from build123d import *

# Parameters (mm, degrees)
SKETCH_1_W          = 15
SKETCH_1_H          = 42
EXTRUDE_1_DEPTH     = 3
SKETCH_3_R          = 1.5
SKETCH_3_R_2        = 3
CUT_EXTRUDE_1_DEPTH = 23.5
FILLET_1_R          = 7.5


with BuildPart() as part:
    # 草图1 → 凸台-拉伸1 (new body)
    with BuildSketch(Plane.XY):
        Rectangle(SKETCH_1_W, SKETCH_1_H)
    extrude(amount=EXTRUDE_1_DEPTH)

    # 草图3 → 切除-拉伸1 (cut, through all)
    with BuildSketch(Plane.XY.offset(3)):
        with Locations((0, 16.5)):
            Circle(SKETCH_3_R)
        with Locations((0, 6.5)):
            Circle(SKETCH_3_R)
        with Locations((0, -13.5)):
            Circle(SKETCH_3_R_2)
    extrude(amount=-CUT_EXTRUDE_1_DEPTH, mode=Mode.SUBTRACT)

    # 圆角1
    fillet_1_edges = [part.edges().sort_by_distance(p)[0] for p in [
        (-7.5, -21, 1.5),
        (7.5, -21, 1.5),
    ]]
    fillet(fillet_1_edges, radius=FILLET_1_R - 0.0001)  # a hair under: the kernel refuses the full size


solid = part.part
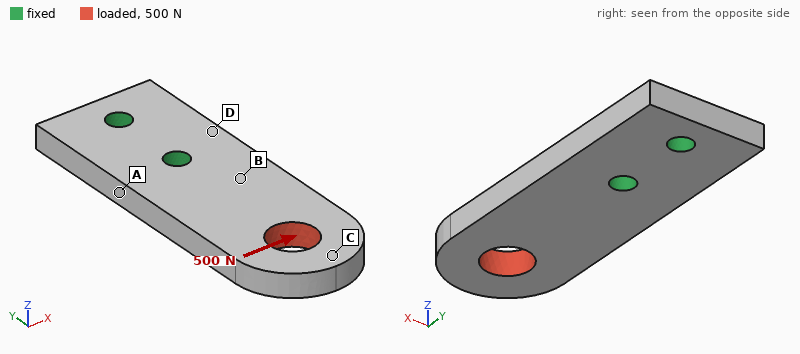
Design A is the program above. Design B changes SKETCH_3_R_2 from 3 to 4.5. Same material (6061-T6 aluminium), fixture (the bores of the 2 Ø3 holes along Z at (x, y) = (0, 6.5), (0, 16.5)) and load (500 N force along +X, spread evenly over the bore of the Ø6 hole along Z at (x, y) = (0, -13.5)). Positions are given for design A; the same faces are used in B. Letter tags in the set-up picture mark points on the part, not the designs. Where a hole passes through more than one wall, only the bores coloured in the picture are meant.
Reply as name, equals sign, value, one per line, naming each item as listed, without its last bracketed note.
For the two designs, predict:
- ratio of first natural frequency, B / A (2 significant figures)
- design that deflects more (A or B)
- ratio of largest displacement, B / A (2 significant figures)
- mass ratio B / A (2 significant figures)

ratio of first natural frequency, B / A = 1.1
design that deflects more = B
ratio of largest displacement, B / A = 1.2
mass ratio B / A = 0.94
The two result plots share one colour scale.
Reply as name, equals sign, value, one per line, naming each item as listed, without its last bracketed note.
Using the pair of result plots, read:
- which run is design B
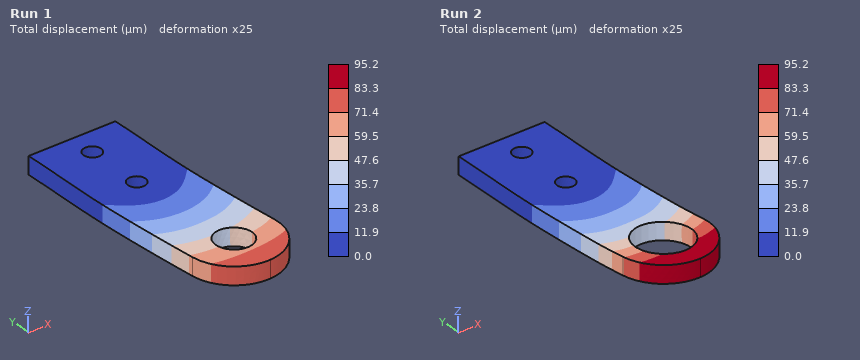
which run is design B = Run 2
